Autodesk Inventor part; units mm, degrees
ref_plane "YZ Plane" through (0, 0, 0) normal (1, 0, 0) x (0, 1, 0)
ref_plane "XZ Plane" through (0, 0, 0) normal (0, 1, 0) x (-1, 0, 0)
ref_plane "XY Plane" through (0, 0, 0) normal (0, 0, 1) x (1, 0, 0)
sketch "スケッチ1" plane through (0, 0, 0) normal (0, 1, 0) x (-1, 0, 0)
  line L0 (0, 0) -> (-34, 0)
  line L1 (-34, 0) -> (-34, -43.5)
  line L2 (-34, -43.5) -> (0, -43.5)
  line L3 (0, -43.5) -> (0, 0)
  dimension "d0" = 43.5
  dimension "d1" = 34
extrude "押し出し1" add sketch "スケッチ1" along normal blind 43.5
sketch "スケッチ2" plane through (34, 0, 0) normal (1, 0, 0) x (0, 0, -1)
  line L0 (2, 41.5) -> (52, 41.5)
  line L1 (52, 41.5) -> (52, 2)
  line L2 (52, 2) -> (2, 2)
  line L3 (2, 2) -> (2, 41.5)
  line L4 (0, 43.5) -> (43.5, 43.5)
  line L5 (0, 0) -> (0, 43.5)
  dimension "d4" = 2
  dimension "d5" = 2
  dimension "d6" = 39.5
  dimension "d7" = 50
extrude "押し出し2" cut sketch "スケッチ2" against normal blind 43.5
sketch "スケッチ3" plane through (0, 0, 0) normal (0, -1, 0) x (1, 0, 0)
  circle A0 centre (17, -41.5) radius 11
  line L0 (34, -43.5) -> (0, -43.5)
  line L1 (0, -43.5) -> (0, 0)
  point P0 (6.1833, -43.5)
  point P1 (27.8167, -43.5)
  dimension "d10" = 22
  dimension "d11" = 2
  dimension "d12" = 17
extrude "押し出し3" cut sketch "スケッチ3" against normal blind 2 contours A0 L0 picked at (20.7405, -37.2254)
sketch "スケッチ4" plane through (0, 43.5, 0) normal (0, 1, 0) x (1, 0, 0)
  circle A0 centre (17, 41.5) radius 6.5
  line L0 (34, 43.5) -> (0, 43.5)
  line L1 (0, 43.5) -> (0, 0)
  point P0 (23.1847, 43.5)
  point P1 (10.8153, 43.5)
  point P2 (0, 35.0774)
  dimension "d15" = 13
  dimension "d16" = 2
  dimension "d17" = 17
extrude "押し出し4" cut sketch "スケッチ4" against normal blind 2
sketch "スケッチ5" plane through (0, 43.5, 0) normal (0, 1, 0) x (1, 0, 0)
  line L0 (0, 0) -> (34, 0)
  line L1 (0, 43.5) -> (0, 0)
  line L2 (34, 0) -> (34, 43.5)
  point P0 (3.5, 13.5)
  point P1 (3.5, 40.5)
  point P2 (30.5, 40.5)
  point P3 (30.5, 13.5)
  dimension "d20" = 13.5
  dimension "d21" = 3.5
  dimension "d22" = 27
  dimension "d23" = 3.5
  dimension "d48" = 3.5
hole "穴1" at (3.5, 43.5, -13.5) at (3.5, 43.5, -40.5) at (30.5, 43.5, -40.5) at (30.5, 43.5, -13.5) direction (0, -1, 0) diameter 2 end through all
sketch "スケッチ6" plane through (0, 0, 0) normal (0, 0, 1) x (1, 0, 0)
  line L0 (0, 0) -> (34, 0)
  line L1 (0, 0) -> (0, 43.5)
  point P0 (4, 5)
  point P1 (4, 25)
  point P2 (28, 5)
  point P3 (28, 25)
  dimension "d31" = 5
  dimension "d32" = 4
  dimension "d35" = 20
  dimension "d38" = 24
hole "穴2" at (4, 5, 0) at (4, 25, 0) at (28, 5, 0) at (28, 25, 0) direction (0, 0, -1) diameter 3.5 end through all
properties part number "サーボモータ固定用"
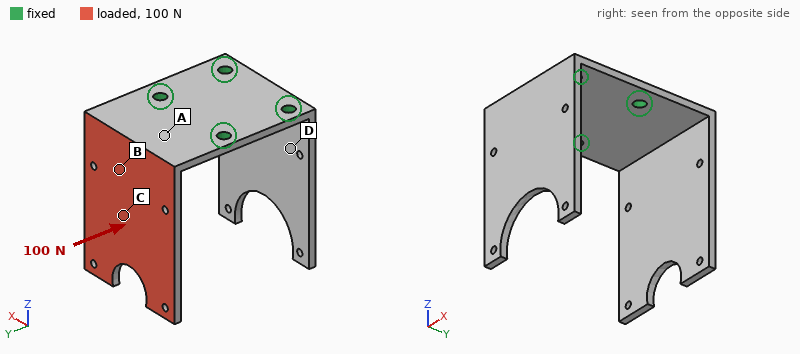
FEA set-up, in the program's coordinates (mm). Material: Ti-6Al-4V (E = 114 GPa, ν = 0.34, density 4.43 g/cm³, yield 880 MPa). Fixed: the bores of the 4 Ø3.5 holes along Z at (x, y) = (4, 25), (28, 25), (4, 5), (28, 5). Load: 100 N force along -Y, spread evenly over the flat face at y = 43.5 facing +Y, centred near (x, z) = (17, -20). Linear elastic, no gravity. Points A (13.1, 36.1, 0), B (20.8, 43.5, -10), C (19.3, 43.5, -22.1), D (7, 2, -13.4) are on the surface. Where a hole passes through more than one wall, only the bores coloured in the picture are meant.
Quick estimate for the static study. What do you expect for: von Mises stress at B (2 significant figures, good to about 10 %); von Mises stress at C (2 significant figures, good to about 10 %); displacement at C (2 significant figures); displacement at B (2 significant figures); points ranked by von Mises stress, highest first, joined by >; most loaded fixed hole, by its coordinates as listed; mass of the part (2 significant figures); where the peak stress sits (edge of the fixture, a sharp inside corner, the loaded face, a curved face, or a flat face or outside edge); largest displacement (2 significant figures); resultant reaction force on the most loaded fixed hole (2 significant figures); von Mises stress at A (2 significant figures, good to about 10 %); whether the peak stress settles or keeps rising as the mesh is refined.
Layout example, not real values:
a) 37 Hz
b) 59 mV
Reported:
a) 46 MPa
b) 17 MPa
c) 0.37 mm
d) 0.18 mm
e) A > B > C > D
f) (28, 25)
g) 35 g
h) edge of the fixture
i) 0.80 mm
j) 48 N
k) 72 MPa
l) keeps rising
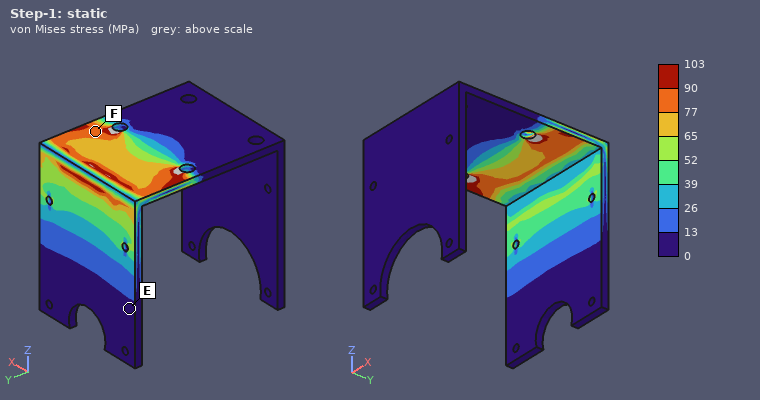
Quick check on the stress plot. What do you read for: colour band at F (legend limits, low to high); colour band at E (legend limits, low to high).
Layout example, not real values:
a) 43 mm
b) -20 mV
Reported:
a) 77 to 90 MPa
b) 0 to 13 MPa
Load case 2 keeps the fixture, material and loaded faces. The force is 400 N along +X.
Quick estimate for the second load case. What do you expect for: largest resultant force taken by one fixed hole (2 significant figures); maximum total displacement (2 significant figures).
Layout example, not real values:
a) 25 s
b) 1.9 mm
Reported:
a) 460 N
b) 0.60 mm
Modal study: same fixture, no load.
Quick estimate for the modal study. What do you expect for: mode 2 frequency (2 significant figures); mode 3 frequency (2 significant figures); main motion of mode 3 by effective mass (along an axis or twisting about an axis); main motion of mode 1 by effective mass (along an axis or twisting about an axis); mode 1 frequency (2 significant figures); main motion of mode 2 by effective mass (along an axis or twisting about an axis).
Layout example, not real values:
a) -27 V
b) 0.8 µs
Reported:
a) 1100 Hz
b) 1400 Hz
c) along X
d) along Y
e) 630 Hz
f) along Y
